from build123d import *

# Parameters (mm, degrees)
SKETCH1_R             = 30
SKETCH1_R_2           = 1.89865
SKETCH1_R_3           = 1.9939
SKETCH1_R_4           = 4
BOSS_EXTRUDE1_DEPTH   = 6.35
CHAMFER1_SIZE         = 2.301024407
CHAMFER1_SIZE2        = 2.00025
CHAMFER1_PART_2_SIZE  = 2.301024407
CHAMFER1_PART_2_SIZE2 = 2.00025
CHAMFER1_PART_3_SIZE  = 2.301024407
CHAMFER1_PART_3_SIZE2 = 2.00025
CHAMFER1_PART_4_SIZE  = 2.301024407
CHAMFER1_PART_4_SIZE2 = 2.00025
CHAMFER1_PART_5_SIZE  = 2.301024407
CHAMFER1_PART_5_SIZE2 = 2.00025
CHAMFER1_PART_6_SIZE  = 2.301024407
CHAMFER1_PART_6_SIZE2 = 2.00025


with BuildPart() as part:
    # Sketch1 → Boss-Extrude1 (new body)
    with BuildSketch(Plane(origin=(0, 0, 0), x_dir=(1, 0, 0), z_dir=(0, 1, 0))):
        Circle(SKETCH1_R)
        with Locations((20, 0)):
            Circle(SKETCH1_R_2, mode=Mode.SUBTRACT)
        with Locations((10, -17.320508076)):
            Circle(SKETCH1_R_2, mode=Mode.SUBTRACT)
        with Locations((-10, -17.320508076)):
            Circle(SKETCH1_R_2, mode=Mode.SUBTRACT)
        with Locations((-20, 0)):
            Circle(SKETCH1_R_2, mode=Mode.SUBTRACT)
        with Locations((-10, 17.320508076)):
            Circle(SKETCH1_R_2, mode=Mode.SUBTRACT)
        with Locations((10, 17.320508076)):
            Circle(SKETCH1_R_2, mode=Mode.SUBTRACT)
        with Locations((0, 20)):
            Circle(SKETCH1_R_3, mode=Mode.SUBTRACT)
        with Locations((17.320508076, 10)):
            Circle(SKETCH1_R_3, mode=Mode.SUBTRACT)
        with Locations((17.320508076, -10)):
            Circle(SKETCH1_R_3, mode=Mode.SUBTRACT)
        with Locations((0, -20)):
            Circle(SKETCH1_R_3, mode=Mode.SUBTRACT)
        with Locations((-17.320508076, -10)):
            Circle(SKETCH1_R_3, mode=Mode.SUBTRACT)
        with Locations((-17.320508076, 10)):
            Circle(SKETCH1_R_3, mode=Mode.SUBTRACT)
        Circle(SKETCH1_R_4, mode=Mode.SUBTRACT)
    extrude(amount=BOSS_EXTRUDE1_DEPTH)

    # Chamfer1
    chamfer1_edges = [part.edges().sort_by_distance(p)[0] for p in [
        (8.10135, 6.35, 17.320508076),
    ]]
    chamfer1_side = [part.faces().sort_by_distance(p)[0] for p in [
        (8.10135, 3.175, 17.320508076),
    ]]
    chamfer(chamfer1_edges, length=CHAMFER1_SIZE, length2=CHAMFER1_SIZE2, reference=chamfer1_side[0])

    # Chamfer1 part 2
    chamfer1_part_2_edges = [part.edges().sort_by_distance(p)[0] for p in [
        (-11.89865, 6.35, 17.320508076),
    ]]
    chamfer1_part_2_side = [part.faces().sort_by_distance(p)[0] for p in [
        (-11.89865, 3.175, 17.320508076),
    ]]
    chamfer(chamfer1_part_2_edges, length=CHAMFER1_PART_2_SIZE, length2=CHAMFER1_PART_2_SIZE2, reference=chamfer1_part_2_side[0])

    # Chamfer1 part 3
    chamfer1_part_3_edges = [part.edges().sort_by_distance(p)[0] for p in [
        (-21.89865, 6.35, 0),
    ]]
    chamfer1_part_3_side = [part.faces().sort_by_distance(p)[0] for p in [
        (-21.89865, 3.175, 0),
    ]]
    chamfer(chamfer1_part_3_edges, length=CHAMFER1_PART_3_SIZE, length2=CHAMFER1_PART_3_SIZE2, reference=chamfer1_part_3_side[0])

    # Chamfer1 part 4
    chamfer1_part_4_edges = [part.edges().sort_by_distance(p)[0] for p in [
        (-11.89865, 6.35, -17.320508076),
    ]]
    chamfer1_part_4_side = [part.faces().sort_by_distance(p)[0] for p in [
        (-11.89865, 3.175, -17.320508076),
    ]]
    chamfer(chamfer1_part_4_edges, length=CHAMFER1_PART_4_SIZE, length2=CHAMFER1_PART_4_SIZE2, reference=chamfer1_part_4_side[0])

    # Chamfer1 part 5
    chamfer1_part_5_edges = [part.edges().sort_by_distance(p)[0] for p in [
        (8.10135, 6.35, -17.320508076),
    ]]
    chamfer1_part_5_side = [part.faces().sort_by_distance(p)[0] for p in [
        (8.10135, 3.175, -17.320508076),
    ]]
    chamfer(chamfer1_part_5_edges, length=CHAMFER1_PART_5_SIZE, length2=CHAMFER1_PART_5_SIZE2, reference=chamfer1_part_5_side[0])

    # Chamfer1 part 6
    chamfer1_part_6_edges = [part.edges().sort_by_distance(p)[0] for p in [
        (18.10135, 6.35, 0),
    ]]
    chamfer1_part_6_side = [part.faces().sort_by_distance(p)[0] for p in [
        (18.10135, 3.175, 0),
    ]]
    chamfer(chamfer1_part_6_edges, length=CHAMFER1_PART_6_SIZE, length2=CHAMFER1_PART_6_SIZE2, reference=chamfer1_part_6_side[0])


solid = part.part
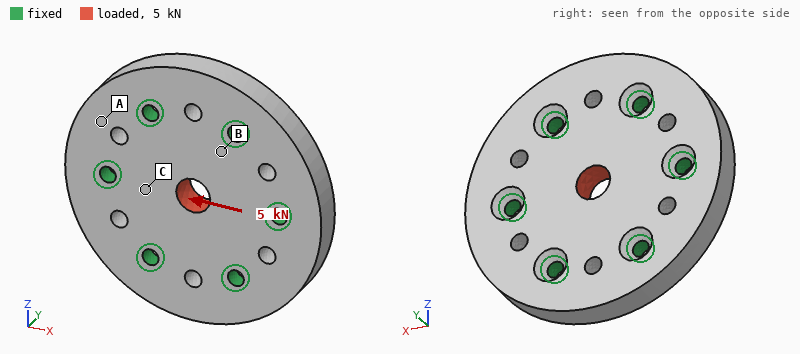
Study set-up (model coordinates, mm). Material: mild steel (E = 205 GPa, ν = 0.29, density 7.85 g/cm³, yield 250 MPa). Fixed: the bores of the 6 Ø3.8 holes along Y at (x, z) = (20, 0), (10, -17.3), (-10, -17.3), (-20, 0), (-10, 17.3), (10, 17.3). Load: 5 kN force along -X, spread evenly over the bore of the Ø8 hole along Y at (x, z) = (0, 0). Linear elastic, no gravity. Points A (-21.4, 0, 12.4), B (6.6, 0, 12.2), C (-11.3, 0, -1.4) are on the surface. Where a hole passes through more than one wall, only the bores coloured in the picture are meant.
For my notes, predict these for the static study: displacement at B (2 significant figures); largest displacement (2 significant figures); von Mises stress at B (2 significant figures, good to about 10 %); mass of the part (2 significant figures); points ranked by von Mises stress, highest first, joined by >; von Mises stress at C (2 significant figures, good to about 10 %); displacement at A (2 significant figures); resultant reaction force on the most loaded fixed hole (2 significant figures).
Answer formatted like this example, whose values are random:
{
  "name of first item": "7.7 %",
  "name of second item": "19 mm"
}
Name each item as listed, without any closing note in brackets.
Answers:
{
  "displacement at B": "0.44 µm",
  "largest displacement": "1.9 µm",
  "von Mises stress at B": "15 MPa",
  "mass of the part": "130 g",
  "points ranked by von Mises stress, highest first, joined by >": "C > B > A",
  "von Mises stress at C": "25 MPa",
  "displacement at A": "0.31 µm",
  "resultant reaction force on the most loaded fixed hole": "1.3 kN"
}
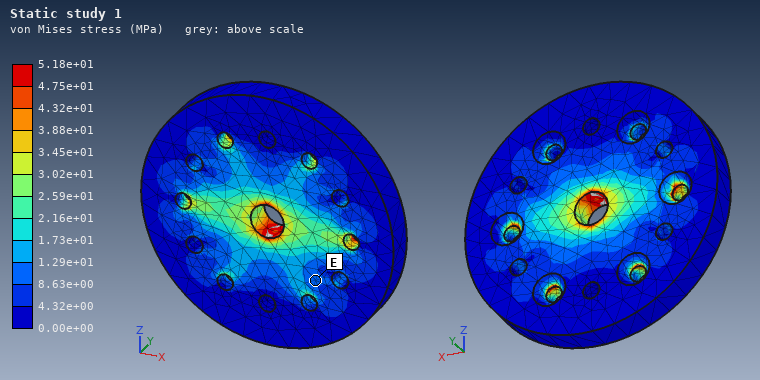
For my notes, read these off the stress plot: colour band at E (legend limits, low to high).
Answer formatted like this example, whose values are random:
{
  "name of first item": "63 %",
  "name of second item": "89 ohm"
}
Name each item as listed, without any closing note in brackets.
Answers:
{
  "colour band at E": "8.63e+00 to 1.29e+01 MPa"
}
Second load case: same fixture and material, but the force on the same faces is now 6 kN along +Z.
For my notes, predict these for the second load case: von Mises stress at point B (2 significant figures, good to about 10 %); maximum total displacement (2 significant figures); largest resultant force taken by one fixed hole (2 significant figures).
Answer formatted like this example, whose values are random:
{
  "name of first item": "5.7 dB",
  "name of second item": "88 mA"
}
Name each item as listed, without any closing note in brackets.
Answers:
{
  "von Mises stress at point B": "28 MPa",
  "maximum total displacement": "2.3 µm",
  "largest resultant force taken by one fixed hole": "1.3 kN"
}
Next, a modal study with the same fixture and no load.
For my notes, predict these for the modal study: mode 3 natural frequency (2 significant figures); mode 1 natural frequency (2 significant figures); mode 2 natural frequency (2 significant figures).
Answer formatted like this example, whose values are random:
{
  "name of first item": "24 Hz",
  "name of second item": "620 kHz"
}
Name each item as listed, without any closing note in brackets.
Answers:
{
  "mode 3 natural frequency": "25 kHz",
  "mode 1 natural frequency": "23 kHz",
  "mode 2 natural frequency": "25 kHz"
}
